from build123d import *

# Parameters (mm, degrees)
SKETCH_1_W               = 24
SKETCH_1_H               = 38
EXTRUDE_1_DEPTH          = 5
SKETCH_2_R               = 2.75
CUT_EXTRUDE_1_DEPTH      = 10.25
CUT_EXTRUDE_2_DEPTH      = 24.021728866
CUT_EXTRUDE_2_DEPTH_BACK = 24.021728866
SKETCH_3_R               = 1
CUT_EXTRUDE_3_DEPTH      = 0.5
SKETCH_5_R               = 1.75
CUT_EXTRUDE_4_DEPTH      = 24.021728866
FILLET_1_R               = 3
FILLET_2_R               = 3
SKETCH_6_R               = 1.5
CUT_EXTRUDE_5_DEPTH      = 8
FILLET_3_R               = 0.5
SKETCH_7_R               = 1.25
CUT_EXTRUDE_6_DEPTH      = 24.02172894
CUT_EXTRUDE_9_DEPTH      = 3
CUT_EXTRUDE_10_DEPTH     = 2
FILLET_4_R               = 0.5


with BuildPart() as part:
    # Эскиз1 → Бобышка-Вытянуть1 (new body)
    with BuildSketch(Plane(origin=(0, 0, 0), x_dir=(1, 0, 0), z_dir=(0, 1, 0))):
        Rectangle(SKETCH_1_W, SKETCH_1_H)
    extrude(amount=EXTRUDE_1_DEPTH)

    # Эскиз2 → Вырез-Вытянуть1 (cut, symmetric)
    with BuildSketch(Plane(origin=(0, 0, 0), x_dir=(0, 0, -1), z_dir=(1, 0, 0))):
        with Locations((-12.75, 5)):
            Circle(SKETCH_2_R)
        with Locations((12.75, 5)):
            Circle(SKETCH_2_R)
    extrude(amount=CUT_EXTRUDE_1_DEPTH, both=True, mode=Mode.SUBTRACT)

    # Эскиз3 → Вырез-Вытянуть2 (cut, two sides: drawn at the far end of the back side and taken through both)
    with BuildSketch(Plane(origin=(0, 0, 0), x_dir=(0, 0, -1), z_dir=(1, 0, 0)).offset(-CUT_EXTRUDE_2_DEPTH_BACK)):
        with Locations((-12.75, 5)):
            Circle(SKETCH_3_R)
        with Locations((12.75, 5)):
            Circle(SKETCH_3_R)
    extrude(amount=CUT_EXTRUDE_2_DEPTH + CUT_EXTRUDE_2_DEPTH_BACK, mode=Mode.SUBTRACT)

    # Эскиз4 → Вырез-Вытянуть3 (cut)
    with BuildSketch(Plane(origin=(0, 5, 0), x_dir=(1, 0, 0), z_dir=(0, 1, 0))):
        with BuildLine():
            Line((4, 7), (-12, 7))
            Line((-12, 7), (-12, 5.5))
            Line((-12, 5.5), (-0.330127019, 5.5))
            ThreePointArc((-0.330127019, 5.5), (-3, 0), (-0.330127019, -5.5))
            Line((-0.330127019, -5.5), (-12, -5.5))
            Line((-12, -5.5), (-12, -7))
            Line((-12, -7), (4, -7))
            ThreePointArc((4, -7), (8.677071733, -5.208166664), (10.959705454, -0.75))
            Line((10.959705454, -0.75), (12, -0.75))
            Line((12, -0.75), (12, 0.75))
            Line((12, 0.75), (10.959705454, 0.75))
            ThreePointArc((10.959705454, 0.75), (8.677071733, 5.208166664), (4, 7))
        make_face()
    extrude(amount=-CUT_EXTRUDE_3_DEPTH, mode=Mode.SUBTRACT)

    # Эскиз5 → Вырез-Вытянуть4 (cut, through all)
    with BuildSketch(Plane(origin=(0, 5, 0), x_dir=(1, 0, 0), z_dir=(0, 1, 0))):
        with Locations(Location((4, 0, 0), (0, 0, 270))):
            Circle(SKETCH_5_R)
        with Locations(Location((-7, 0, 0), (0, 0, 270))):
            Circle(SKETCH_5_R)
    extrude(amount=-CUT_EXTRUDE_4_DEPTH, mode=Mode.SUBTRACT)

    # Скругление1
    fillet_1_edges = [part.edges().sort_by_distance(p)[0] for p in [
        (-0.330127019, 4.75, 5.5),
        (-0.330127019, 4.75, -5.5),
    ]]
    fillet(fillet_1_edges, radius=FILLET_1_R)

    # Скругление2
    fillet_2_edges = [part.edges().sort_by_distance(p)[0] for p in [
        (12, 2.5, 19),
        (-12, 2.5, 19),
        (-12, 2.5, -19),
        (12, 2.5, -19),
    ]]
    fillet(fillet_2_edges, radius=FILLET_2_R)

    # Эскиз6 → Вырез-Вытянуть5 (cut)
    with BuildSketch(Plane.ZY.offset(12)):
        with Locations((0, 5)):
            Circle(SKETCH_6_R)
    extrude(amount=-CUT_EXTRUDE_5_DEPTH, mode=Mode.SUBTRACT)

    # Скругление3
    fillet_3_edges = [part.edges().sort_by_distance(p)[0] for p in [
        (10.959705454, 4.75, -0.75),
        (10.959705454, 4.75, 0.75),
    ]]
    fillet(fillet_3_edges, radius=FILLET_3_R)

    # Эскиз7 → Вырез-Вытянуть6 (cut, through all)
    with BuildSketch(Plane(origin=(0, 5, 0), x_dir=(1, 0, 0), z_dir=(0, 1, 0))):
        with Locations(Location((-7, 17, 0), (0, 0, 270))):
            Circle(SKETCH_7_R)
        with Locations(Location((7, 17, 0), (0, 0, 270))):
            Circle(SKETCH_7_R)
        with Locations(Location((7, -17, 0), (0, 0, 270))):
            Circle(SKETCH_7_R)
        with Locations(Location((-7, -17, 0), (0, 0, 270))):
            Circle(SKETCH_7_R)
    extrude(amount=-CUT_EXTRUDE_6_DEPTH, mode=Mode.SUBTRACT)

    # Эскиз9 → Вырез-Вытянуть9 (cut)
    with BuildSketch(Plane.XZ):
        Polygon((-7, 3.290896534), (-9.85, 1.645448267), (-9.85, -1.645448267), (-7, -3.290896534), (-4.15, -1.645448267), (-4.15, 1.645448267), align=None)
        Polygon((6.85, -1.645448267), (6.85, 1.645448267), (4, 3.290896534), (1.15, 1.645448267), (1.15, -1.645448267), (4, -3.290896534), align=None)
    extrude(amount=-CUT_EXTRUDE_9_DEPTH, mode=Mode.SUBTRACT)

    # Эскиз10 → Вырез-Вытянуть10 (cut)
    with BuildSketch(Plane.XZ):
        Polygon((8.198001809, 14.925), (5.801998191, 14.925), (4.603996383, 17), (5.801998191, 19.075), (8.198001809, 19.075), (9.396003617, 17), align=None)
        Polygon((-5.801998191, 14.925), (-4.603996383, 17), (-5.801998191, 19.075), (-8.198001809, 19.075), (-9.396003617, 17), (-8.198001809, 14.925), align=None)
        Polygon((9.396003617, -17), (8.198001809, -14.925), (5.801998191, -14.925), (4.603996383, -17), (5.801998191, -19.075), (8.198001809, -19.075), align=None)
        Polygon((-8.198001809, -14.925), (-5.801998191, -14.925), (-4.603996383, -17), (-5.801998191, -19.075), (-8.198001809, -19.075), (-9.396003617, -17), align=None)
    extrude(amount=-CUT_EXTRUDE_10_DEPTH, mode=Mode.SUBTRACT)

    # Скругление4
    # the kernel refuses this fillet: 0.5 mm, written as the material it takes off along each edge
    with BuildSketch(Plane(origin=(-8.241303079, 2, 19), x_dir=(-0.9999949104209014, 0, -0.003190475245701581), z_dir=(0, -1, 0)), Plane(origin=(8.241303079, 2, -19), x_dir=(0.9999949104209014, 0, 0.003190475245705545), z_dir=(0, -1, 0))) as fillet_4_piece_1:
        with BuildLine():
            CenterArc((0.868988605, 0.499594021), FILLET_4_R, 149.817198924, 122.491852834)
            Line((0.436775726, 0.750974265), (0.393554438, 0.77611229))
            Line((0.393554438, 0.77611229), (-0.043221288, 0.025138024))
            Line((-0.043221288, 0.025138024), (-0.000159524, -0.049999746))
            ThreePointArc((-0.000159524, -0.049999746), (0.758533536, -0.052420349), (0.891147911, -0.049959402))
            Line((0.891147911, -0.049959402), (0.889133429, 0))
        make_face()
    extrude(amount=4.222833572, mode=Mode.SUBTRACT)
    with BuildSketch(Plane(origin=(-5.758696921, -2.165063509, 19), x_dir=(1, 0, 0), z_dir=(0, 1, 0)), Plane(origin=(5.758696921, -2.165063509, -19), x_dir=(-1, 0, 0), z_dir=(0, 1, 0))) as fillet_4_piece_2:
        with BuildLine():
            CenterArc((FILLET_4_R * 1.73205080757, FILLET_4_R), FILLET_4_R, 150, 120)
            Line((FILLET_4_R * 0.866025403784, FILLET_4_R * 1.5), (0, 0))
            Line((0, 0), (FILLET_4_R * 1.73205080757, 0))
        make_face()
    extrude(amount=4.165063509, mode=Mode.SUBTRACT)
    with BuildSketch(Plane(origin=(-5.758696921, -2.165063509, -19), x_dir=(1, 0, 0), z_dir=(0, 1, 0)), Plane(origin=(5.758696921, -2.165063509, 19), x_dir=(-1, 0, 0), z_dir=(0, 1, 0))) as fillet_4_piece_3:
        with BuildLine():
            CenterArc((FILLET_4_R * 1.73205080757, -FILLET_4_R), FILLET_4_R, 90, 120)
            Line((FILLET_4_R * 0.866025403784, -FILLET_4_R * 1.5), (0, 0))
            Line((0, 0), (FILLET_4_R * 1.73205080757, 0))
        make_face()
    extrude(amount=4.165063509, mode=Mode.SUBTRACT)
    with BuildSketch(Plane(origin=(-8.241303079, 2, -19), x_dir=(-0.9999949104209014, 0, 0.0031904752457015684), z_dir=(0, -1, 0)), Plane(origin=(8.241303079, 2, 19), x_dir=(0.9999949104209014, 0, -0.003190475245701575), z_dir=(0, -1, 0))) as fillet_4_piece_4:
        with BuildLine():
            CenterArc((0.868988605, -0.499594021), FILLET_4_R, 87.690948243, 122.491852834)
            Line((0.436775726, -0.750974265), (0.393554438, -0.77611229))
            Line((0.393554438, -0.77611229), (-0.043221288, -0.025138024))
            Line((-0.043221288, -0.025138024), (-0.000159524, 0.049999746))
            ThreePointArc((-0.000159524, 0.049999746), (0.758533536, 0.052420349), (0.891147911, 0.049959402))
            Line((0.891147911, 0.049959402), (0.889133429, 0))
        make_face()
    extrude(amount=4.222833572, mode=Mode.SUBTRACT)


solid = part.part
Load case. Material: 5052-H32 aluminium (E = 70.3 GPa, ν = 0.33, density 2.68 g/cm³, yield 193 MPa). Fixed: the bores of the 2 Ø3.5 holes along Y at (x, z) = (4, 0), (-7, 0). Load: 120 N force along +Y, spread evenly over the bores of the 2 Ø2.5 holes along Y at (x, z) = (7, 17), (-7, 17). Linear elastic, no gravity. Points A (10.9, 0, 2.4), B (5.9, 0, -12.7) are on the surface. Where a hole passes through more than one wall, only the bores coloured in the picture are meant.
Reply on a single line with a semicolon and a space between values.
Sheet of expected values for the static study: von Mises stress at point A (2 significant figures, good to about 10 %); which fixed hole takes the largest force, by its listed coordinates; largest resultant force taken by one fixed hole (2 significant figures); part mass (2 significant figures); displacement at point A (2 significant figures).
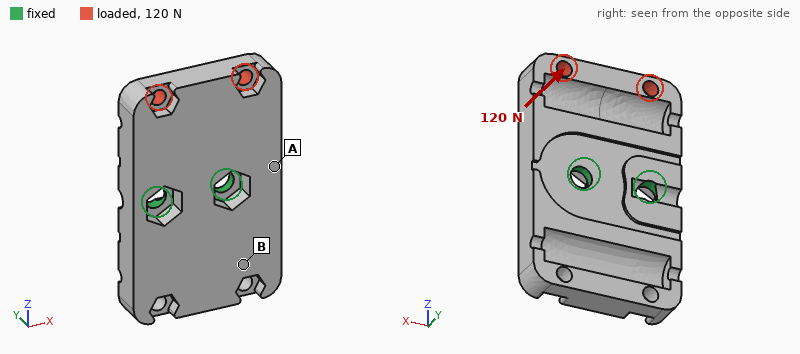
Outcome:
20 MPa; (4, 0); 73 N; 9.4 g; 7.7 µm
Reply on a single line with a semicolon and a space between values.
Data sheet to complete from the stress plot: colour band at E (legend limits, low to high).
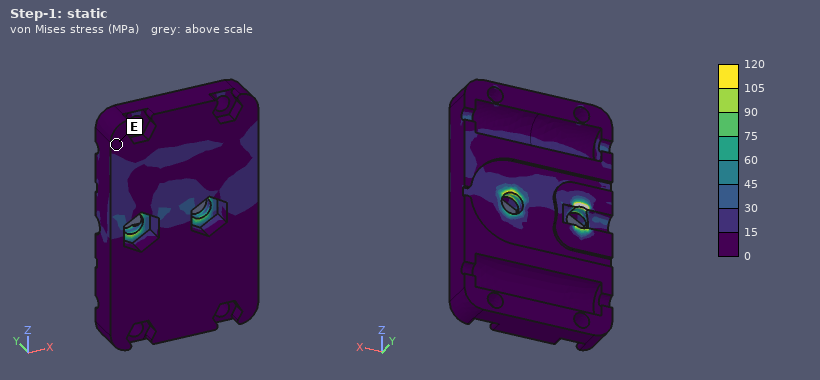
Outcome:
0 to 15 MPa
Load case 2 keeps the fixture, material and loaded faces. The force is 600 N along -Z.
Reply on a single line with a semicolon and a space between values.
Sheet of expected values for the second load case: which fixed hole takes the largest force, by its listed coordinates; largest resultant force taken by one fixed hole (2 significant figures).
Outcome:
(4, 0); 370 N
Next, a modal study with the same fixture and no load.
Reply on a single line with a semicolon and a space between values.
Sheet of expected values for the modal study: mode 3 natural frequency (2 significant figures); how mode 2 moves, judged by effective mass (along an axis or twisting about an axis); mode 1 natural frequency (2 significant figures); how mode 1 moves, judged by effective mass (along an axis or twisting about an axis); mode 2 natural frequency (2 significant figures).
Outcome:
14 kHz; along Y; 5400 Hz; twisting about X; 10 kHz
